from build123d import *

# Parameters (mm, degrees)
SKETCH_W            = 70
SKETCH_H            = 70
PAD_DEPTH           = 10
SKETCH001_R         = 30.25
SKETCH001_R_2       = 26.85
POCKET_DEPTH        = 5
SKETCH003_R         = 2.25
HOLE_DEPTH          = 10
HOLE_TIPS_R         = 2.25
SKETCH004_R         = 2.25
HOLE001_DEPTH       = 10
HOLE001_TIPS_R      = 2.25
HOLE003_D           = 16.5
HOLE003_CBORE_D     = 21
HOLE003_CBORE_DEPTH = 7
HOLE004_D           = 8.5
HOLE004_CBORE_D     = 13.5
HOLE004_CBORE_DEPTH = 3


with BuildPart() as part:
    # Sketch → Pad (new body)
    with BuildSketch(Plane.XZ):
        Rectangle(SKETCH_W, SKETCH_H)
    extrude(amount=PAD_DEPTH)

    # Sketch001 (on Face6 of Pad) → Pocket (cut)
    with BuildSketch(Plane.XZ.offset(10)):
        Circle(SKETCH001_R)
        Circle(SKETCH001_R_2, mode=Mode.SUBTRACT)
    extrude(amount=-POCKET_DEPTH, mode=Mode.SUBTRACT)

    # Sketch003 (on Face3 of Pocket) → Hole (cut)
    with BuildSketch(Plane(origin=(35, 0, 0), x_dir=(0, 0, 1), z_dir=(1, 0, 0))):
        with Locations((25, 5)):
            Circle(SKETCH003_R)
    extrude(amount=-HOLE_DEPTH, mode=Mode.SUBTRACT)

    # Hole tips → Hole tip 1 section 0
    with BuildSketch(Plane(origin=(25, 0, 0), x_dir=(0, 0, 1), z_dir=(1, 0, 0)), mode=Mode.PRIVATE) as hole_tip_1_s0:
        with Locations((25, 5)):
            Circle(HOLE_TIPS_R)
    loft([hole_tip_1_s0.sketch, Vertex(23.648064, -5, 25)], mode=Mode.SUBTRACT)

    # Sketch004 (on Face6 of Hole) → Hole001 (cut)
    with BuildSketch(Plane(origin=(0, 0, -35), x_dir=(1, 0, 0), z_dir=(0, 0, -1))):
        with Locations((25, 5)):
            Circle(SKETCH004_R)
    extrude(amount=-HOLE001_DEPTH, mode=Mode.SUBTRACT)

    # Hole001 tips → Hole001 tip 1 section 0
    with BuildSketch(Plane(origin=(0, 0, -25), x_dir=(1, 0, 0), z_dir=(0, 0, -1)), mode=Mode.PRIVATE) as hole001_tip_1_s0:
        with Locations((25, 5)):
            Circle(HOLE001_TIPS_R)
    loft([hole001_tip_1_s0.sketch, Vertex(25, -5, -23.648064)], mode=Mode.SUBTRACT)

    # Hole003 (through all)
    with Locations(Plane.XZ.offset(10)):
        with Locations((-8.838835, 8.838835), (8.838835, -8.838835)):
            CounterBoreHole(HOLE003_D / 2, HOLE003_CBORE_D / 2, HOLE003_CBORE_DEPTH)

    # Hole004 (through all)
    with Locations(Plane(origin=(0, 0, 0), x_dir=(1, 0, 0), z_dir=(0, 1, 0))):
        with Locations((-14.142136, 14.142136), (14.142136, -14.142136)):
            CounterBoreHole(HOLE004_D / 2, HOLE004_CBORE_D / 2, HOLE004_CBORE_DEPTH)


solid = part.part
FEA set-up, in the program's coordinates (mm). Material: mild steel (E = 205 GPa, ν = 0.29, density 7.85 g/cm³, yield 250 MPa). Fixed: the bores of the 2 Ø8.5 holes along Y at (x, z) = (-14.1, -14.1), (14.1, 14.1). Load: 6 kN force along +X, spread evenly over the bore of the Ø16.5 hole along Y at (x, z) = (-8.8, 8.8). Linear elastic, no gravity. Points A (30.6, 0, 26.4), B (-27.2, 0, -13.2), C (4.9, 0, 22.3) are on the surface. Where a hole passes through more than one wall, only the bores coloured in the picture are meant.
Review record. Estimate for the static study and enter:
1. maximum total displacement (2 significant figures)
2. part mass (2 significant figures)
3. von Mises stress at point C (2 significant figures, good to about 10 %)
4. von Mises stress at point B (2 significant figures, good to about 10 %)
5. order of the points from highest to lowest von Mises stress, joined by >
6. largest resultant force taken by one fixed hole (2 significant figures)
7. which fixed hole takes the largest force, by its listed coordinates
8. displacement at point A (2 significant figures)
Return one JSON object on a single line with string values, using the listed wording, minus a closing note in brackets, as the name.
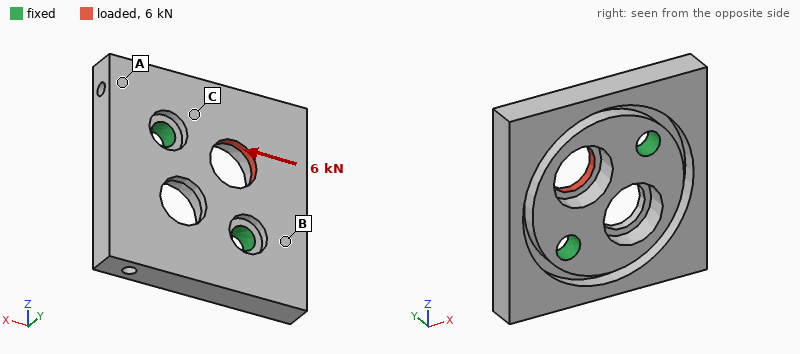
{"maximum total displacement": "19 µm", "part mass": "300 g", "von Mises stress at point C": "24 MPa", "von Mises stress at point B": "13 MPa", "order of the points from highest to lowest von Mises stress, joined by >": "C > B > A", "largest resultant force taken by one fixed hole": "4.0 kN", "which fixed hole takes the largest force, by its listed coordinates": "(14.1, 14.1)", "displacement at point A": "3.3 µm"}
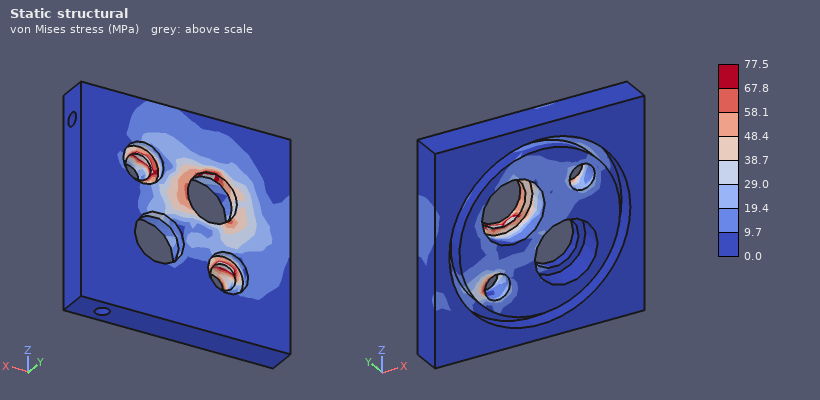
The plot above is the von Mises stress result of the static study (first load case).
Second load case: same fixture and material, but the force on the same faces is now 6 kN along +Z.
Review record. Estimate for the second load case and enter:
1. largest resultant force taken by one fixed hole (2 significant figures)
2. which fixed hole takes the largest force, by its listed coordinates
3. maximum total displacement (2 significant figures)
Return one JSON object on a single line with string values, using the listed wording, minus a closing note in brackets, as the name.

{"largest resultant force taken by one fixed hole": "4.0 kN", "which fixed hole takes the largest force, by its listed coordinates": "(-14.1, -14.1)", "maximum total displacement": "19 µm"}
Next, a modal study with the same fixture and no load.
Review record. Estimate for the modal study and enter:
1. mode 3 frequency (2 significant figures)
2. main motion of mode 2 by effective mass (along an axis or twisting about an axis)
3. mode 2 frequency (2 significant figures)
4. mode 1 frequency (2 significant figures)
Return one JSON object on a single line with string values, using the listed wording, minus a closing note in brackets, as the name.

{"mode 3 frequency": "7800 Hz", "main motion of mode 2 by effective mass": "along Y", "mode 2 frequency": "4500 Hz", "mode 1 frequency": "3900 Hz"}
